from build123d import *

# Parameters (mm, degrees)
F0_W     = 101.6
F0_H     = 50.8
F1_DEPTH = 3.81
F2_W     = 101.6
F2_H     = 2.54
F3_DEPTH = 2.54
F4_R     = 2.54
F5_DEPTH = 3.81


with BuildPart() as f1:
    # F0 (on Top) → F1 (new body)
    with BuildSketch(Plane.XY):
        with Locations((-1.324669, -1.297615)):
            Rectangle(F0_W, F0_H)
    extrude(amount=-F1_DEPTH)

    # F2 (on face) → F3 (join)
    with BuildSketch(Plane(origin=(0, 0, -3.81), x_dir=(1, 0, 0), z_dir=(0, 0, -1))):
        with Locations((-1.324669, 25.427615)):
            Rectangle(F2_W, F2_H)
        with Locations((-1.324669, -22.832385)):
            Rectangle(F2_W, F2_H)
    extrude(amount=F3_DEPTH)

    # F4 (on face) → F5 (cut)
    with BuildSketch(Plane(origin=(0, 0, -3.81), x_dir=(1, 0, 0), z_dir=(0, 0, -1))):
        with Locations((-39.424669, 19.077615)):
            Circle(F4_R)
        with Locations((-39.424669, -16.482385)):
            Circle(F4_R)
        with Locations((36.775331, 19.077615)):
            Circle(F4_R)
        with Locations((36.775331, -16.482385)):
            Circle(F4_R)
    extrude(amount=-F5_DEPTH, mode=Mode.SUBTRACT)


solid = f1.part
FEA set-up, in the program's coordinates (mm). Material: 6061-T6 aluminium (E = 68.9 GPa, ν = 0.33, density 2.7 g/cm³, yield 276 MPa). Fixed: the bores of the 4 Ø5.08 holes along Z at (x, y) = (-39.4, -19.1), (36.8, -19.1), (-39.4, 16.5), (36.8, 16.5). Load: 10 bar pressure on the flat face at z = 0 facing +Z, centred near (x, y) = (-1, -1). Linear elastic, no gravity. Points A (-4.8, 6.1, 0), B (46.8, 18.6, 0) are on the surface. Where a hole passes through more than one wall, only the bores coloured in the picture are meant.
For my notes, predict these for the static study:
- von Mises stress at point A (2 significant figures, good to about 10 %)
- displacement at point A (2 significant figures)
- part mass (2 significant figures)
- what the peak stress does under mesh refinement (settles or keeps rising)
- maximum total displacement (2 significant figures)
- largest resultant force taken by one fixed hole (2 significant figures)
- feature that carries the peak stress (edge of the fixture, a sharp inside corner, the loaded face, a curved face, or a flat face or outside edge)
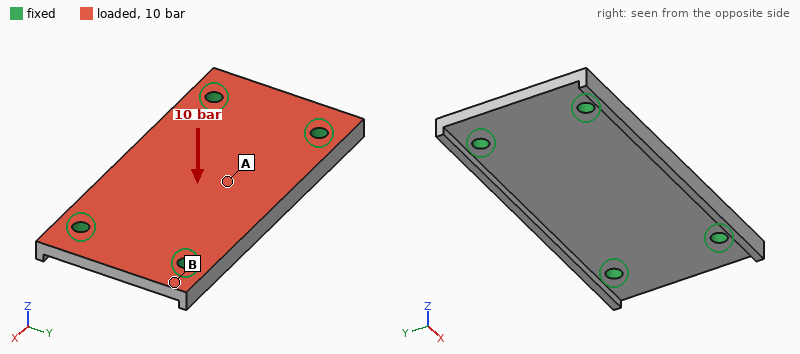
67 MPa
0.21 mm
56 g
keeps rising
0.22 mm
1.3 kN
edge of the fixture
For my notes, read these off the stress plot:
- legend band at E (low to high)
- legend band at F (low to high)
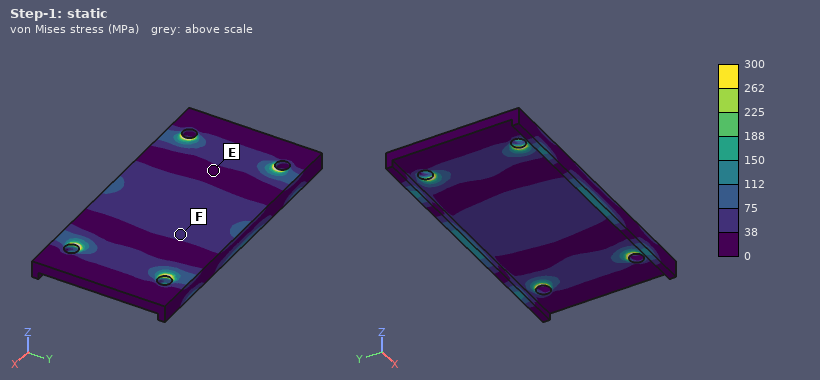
0 to 38 MPa
38 to 75 MPa
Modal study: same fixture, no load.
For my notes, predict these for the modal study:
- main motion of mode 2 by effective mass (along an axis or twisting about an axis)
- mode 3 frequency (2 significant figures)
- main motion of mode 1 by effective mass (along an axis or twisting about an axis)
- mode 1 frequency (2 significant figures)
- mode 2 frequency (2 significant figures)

twisting about X
9600 Hz
along Z
3800 Hz
5300 Hz
